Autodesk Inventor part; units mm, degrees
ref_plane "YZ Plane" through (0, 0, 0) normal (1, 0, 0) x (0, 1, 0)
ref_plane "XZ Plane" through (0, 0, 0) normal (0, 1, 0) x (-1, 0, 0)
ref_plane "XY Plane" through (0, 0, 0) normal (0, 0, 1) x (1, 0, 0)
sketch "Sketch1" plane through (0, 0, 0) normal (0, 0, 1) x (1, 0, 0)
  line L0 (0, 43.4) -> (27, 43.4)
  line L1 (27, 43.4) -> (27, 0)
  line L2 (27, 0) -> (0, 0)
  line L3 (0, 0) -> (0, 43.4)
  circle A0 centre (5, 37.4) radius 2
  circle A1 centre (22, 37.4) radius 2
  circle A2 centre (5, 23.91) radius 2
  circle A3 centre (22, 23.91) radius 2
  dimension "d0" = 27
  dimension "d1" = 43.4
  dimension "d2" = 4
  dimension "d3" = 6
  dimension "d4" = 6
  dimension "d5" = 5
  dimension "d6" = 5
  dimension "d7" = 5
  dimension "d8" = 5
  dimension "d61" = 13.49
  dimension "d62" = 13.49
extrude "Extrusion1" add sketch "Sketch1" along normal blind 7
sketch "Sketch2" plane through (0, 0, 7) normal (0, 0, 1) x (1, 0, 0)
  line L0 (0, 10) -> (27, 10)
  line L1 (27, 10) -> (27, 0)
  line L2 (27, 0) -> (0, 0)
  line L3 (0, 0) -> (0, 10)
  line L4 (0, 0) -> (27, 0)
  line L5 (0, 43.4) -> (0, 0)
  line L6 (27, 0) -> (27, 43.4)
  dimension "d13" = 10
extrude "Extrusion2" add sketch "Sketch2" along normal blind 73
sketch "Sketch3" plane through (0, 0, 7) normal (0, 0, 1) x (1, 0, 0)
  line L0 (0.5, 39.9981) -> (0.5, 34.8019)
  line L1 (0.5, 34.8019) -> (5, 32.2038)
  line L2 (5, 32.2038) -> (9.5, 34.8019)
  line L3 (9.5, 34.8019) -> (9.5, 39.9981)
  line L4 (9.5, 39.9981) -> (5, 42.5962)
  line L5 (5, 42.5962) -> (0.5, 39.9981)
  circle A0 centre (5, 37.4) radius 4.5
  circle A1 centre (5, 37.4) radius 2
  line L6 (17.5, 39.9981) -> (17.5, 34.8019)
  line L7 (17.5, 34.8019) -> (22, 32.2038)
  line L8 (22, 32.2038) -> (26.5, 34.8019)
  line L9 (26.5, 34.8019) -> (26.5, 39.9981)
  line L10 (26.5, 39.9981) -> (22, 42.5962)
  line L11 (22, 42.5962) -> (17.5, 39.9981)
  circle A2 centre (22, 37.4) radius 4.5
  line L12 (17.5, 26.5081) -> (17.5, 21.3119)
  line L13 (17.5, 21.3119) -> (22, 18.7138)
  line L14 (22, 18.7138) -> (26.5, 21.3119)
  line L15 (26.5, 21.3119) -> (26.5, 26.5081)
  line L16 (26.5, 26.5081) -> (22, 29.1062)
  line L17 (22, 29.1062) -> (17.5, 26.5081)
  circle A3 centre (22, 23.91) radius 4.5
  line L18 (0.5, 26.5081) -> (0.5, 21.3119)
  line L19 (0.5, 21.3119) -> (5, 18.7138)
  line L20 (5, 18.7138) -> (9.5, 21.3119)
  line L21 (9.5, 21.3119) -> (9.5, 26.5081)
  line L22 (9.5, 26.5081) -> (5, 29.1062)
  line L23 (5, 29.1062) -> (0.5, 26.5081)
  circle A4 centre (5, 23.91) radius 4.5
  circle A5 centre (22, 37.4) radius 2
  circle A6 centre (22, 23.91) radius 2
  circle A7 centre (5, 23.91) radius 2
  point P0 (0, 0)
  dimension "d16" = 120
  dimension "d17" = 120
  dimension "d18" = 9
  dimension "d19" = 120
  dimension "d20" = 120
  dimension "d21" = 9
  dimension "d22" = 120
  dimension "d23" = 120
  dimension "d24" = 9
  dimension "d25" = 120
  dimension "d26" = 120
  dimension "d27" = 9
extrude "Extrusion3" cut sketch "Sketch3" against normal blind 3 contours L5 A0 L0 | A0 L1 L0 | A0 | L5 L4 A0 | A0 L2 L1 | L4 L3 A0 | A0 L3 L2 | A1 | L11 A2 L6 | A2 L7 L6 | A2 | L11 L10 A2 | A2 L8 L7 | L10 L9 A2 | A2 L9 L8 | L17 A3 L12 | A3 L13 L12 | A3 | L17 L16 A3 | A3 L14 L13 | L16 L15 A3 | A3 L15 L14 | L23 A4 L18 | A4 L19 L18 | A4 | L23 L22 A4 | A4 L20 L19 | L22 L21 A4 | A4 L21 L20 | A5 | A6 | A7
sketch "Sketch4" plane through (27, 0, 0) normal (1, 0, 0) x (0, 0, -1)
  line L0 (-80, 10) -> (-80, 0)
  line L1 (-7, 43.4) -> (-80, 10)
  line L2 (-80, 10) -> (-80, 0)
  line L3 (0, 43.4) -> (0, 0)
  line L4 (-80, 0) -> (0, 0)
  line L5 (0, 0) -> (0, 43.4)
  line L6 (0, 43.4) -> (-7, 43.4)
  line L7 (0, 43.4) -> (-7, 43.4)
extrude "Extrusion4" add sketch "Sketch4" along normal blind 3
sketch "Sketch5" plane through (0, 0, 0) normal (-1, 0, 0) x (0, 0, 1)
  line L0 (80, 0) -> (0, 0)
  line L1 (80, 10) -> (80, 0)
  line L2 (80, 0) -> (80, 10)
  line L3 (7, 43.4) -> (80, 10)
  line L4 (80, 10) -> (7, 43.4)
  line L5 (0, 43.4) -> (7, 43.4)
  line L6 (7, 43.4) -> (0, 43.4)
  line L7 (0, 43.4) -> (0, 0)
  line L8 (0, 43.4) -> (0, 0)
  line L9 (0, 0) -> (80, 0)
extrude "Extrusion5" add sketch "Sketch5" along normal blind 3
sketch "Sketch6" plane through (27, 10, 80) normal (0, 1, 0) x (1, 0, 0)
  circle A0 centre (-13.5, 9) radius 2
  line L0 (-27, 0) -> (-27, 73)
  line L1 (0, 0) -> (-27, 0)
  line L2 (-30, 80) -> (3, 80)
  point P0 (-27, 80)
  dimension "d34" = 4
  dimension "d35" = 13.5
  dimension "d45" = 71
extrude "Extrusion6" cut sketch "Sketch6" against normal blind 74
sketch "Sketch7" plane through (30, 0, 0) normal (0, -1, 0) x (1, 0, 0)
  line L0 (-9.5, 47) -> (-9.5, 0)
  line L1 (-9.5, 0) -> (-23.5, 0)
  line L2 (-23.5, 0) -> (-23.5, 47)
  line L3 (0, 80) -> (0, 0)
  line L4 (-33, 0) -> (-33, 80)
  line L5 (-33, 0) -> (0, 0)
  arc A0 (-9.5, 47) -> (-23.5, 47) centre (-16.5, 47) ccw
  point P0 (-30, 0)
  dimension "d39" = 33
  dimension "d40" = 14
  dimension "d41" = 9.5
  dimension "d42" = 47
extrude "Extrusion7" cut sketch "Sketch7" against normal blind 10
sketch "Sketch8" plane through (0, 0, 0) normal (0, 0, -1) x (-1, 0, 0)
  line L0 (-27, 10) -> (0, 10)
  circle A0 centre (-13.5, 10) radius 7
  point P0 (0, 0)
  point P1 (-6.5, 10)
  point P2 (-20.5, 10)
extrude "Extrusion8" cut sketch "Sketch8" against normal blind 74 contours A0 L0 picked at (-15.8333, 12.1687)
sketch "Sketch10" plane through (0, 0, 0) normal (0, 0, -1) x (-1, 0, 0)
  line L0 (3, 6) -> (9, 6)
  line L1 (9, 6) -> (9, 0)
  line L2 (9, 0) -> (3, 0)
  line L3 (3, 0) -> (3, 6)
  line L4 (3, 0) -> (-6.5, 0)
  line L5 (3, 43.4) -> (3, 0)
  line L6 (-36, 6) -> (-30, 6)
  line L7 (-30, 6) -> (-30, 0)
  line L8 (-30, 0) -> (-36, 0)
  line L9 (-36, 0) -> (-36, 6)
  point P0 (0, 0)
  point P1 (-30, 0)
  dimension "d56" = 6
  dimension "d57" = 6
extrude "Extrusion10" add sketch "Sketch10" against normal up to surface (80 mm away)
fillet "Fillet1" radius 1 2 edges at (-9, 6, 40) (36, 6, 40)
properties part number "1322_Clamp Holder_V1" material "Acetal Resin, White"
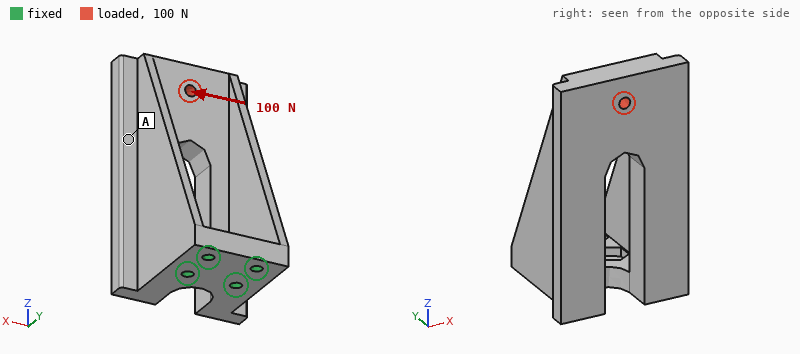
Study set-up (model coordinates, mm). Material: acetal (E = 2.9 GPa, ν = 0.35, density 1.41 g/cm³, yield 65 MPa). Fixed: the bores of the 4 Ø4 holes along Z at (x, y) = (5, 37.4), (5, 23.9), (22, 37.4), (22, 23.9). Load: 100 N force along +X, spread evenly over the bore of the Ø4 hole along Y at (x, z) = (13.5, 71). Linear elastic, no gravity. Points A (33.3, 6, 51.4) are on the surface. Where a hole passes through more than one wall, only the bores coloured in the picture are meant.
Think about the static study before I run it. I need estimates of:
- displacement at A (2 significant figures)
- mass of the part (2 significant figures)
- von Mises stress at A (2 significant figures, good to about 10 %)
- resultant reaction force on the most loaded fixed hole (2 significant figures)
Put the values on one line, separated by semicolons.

0.76 mm; 54 g; 2.0 MPa; 270 N
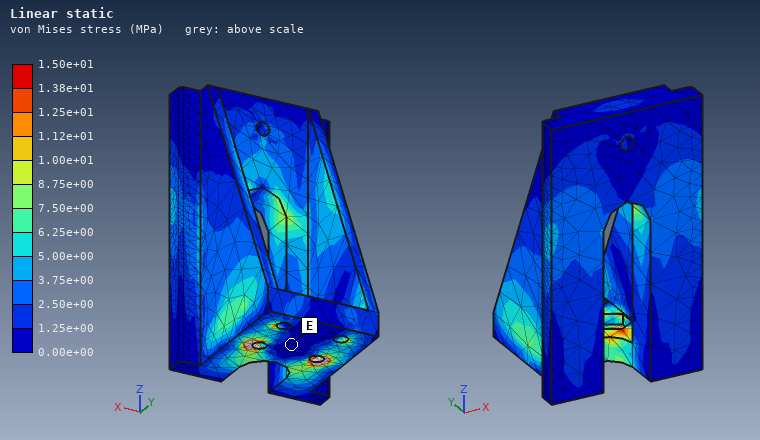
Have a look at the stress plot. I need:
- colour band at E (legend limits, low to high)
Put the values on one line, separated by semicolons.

0.00e+00 to 1.25e+00 MPa
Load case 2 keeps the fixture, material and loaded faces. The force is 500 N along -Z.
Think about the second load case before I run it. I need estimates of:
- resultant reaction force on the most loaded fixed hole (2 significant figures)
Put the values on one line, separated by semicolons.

500 N
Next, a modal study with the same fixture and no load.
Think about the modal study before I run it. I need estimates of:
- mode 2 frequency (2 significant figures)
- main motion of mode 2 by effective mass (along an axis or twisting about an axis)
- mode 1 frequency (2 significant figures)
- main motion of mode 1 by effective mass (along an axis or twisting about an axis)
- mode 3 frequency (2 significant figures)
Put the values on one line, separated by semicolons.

450 Hz; along Y; 350 Hz; along X; 1000 Hz
